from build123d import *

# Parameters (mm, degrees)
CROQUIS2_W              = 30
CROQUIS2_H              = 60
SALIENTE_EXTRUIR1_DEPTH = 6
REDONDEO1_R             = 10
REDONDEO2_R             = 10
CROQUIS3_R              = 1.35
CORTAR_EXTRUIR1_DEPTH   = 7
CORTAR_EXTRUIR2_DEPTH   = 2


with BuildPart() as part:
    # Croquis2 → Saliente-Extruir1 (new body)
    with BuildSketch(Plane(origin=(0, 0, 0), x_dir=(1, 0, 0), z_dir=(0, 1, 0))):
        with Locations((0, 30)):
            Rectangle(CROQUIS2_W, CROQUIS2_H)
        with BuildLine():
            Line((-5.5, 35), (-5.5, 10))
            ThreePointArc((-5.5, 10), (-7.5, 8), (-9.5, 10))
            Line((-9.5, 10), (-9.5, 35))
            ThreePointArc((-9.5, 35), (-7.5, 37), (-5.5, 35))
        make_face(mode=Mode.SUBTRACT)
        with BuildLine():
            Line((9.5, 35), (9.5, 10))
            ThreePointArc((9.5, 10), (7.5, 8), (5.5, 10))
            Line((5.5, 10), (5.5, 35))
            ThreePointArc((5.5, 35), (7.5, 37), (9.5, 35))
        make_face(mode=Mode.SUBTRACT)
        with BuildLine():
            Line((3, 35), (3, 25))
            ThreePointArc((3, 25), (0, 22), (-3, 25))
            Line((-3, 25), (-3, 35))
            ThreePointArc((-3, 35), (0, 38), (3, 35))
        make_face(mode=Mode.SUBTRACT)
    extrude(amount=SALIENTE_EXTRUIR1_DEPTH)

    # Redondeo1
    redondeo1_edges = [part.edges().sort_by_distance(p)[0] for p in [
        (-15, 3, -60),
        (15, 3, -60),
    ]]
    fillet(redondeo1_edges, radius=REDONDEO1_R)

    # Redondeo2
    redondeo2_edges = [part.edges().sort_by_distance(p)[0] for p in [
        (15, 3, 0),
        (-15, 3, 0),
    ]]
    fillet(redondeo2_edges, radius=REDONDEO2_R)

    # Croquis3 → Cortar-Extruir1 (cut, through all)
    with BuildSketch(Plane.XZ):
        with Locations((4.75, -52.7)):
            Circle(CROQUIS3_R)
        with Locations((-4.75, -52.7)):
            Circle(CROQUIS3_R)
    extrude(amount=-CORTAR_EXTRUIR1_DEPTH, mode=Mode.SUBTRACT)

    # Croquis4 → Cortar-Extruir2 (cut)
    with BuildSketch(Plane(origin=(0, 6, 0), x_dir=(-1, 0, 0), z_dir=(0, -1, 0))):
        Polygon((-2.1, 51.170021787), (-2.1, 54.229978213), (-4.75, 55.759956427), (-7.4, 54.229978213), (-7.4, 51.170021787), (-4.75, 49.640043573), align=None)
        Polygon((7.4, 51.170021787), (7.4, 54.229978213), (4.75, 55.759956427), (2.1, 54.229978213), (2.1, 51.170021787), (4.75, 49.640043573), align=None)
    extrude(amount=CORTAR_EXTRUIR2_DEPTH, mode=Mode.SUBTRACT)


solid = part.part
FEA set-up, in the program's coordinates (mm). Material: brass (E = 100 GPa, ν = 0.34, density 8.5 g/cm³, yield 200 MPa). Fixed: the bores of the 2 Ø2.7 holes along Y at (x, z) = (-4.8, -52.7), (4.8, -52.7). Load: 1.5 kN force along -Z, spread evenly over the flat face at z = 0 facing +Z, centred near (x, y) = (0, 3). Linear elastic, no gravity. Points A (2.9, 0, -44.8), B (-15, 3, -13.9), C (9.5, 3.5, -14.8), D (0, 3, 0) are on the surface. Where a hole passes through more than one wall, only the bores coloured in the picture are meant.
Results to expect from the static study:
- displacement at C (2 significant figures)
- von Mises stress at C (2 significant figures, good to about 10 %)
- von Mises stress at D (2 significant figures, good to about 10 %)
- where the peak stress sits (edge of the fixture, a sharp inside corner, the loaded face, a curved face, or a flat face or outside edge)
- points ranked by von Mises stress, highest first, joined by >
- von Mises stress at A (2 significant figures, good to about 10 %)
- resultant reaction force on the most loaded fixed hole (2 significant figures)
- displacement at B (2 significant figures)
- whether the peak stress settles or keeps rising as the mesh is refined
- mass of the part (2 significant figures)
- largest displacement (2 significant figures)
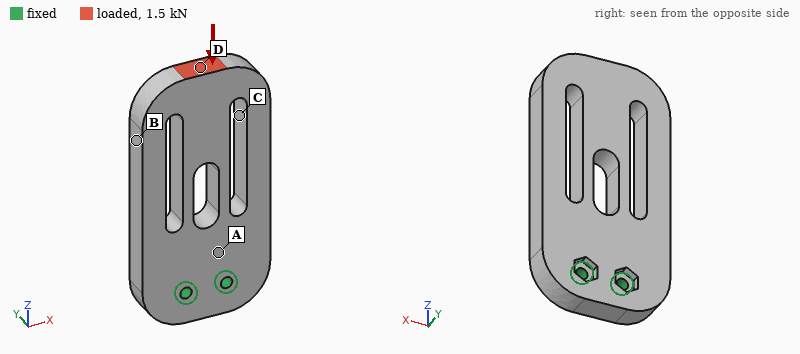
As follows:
11 µm
20 MPa
29 MPa
edge of the fixture
D > C > A > B
11 MPa
750 N
11 µm
keeps rising
70 g
18 µm
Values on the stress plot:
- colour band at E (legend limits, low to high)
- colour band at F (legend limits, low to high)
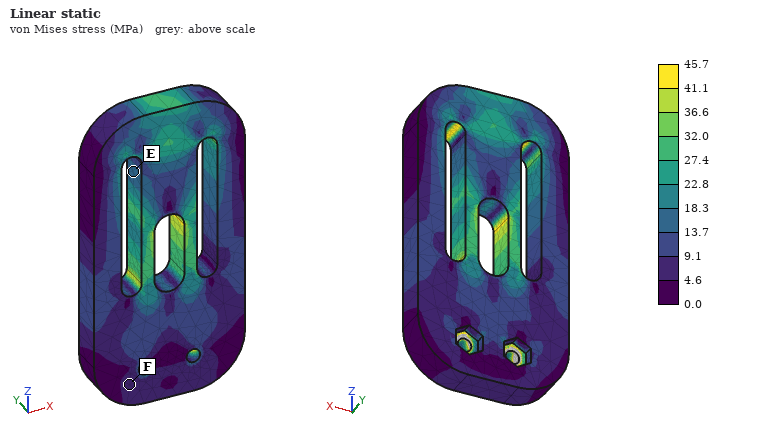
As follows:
13.7 to 18.3 MPa
4.6 to 9.1 MPa
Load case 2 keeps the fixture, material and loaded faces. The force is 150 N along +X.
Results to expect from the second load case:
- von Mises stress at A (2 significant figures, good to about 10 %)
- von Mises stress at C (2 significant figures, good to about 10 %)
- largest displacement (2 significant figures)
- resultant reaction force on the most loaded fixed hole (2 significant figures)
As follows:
8.9 MPa
12 MPa
31 µm
700 N
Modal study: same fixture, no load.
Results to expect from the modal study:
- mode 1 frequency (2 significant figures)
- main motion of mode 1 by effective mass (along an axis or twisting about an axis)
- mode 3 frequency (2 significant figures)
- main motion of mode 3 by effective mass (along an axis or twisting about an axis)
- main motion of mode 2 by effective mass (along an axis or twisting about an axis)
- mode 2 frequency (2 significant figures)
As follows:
1000 Hz
along Y
3200 Hz
twisting about Z
along X
2400 Hz
